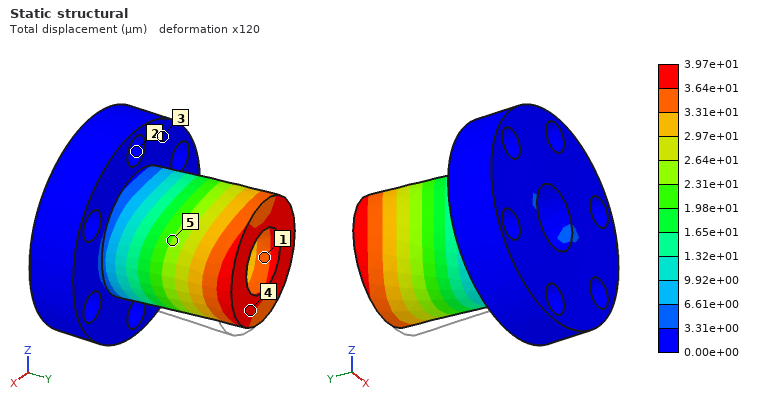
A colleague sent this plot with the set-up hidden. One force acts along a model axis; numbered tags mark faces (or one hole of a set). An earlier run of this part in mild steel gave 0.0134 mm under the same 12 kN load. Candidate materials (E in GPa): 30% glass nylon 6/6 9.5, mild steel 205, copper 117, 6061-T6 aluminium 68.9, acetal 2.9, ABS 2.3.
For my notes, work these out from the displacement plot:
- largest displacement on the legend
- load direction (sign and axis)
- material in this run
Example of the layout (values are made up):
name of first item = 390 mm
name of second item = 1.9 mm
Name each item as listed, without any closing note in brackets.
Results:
largest displacement on the legend = 3.97e+01 µm
load direction = -X
material in this run = 6061-T6 aluminium
